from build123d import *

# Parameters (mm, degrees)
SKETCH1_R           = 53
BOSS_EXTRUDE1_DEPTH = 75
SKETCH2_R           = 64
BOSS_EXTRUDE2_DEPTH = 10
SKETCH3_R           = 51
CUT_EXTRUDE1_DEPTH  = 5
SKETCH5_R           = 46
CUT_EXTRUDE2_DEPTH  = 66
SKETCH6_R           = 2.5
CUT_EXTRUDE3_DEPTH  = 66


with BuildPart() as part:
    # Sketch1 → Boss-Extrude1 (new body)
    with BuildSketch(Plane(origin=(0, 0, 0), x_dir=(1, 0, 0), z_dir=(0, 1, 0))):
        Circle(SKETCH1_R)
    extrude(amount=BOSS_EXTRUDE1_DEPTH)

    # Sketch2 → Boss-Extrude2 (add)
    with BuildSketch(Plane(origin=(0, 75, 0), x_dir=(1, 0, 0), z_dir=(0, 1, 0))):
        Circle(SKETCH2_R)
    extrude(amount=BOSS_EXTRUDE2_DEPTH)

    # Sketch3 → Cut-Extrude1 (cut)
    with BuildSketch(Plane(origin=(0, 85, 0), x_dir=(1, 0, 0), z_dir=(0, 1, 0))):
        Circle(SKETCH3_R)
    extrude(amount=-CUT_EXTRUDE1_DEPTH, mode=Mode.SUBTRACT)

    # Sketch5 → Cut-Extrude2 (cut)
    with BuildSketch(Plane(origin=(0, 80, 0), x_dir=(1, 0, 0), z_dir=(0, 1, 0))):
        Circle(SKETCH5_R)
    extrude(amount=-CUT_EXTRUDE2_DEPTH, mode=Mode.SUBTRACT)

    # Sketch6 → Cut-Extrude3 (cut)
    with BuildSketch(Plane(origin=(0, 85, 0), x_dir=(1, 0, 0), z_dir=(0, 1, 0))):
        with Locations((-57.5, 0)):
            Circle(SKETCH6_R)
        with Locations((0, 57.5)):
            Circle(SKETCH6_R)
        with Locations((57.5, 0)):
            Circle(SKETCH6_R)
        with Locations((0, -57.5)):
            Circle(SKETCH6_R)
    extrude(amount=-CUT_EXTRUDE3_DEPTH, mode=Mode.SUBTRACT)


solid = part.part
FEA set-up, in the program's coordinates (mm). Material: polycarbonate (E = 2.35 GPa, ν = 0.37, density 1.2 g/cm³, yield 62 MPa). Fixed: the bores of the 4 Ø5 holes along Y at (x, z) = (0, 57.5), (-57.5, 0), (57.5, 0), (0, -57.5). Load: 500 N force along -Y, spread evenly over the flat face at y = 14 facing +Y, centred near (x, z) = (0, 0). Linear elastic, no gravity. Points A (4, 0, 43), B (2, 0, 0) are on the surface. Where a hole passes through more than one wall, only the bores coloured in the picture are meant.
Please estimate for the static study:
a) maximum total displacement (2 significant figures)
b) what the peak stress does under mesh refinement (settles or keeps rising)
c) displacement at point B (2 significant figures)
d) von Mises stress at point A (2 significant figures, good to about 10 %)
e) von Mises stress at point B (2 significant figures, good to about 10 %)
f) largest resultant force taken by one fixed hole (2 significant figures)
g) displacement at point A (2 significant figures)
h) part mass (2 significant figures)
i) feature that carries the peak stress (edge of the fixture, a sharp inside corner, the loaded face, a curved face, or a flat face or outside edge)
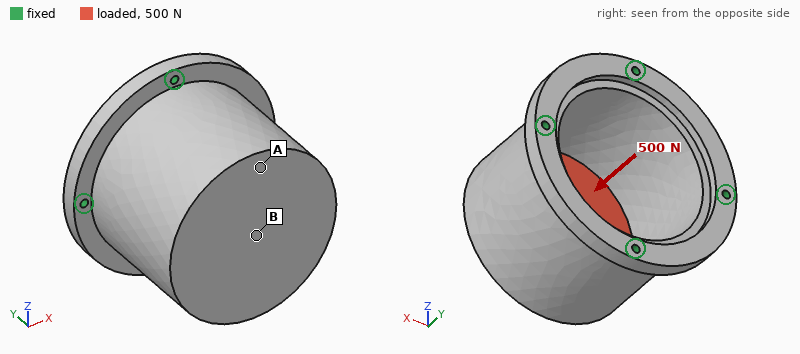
50 µm
keeps rising
50 µm
0.33 MPa
0.87 MPa
130 N
25 µm
370 g
edge of the fixture
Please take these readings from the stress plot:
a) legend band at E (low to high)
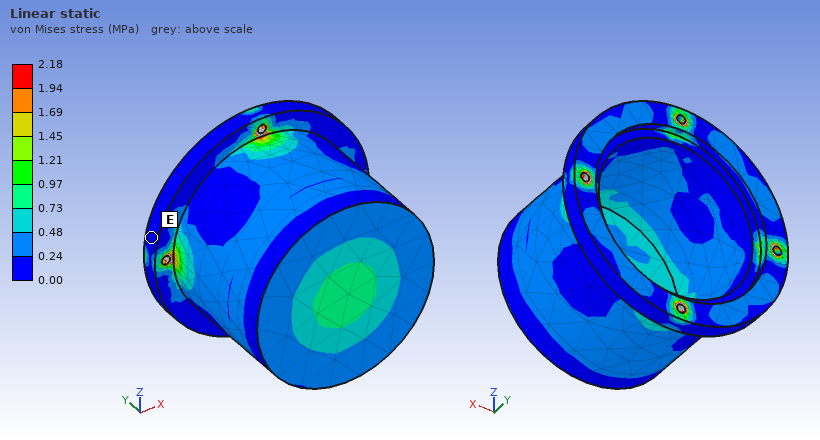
0.00 to 0.24 MPa
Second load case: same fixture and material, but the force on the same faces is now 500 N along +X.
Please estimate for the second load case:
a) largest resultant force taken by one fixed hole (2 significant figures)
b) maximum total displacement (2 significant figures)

310 N
0.10 mm
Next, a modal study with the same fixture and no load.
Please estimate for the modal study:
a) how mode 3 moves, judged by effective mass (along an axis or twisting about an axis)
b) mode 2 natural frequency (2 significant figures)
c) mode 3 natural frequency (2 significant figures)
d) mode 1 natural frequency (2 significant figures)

along Y
780 Hz
1400 Hz
780 Hz
